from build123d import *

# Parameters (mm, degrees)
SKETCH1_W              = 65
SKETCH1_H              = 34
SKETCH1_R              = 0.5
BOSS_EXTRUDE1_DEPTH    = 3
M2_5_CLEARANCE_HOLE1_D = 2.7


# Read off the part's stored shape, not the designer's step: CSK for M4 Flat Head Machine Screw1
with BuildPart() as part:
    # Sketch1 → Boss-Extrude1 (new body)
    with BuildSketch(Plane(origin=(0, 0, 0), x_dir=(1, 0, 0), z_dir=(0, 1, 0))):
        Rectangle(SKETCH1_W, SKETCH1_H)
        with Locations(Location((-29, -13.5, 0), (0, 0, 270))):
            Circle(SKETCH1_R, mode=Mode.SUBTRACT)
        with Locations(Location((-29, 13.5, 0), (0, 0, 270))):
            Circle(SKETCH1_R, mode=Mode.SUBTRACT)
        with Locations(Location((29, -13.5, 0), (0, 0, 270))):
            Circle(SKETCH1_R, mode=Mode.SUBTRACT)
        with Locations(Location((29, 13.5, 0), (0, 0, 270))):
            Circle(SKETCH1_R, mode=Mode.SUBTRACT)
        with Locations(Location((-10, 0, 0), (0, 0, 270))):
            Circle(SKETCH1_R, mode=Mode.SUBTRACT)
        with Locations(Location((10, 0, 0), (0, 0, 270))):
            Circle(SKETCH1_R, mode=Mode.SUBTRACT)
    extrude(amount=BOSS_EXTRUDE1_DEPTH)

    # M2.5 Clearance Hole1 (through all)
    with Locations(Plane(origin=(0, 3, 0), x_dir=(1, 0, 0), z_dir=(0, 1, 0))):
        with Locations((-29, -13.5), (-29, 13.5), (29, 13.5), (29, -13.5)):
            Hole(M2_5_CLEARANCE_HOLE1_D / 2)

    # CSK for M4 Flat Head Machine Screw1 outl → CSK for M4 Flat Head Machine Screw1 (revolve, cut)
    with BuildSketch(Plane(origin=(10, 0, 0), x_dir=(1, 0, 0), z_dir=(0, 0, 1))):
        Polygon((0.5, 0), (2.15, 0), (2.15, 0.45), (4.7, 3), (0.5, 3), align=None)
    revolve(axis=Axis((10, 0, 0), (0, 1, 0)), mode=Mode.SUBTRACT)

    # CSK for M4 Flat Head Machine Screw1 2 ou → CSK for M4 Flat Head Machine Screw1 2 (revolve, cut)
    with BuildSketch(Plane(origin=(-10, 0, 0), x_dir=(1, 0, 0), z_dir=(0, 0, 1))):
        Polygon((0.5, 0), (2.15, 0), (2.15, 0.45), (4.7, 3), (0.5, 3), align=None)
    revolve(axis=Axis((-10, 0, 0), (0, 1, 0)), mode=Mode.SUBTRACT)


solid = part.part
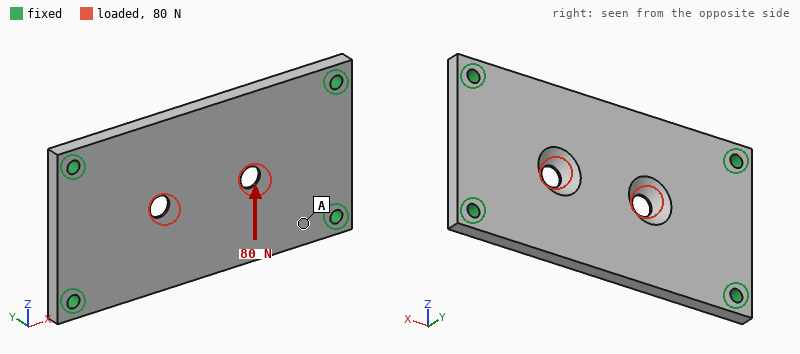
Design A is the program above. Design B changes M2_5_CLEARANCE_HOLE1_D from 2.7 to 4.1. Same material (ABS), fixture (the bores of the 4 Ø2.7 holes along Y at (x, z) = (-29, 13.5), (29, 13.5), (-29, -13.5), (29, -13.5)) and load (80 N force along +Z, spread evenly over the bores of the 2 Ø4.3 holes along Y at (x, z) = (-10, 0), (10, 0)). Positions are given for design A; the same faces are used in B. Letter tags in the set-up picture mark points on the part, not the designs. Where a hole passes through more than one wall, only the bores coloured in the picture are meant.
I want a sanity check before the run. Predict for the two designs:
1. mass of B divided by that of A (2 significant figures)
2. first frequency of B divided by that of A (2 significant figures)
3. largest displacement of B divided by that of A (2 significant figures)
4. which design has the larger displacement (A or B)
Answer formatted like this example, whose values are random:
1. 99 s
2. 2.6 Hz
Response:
1. 0.99
2. 1.1
3. 0.92
4. A
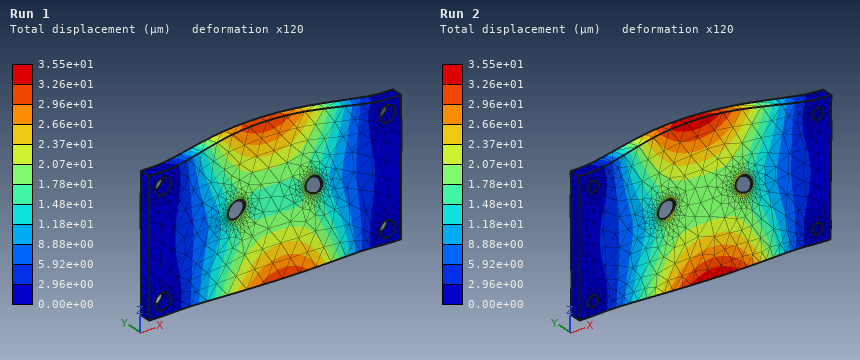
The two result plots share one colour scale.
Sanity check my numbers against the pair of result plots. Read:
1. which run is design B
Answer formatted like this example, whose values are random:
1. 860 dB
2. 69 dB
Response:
1. Run 1
